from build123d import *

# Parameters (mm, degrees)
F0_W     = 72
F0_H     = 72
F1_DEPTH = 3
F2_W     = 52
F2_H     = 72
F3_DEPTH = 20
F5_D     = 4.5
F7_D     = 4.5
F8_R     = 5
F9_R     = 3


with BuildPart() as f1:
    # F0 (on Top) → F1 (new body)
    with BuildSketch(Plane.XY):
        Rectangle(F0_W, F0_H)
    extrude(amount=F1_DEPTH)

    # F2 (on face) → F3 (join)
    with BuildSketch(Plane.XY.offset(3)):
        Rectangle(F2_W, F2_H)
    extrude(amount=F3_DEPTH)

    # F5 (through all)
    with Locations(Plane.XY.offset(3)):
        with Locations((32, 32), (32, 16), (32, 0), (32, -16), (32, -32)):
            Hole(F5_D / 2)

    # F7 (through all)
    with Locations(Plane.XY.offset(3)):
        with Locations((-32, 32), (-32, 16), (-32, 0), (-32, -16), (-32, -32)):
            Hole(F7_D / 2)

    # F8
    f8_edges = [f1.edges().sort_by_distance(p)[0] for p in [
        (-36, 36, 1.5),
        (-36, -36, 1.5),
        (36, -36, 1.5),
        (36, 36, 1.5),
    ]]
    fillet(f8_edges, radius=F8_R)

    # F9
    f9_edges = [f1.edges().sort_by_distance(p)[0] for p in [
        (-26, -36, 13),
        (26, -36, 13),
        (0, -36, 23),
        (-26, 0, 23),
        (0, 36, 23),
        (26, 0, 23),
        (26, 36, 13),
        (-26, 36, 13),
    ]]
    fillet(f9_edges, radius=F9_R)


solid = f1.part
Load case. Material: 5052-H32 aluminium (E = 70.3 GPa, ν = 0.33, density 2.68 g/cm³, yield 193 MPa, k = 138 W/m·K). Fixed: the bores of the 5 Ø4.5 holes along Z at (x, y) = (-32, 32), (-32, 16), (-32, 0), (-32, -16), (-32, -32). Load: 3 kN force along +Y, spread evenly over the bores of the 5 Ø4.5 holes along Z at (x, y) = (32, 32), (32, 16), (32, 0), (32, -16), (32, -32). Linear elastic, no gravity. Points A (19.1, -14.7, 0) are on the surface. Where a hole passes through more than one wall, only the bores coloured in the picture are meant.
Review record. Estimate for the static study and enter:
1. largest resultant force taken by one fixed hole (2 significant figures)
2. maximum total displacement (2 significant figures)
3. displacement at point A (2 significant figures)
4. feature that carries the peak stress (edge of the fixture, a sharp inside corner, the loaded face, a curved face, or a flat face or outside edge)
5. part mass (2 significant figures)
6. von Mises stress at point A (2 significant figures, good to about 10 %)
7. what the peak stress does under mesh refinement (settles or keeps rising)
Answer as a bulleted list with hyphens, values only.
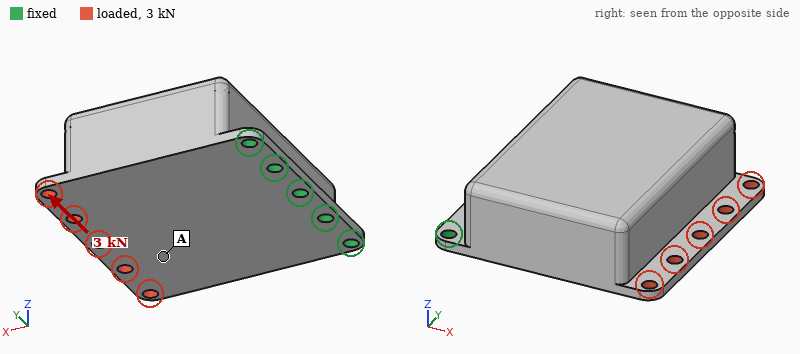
- 2.4 kN
- 64 µm
- 37 µm
- edge of the fixture
- 240 g
- 13 MPa
- keeps rising
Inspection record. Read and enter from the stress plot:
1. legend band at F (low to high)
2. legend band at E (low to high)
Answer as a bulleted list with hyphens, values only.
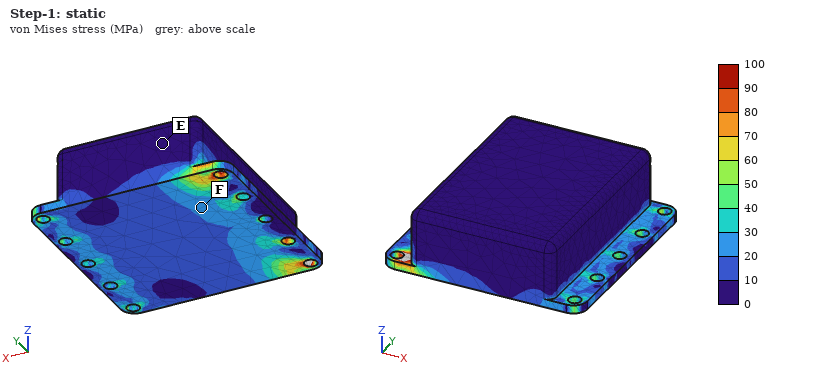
- 20 to 30 MPa
- 0 to 10 MPa
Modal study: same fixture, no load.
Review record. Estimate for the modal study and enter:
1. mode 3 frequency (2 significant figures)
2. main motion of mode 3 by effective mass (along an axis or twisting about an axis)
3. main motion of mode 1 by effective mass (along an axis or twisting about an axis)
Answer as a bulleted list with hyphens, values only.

- 4800 Hz
- along Y
- along Z
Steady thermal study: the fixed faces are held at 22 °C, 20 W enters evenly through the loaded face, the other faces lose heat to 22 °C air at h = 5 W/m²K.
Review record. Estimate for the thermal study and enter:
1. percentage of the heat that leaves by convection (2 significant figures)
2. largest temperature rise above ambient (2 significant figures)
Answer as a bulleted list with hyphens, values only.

- 3.1 %
- 21 K
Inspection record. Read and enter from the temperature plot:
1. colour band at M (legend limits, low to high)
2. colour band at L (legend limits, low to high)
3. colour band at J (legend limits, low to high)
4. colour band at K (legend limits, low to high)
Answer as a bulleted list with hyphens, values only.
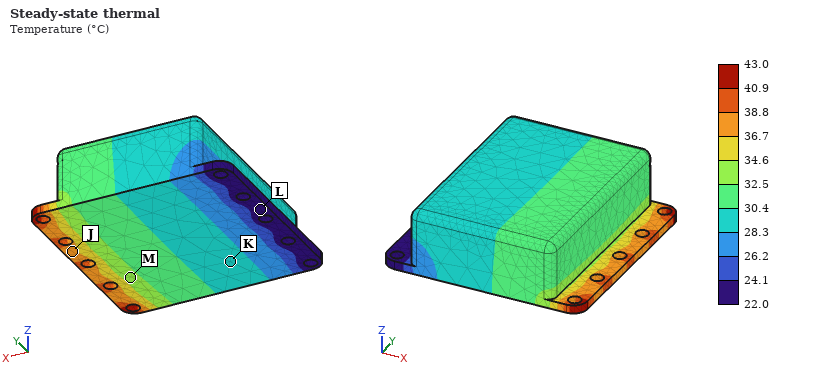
- 32.5 to 34.6 °C
- 22.0 to 24.1 °C
- 36.7 to 38.8 °C
- 28.3 to 30.4 °C
